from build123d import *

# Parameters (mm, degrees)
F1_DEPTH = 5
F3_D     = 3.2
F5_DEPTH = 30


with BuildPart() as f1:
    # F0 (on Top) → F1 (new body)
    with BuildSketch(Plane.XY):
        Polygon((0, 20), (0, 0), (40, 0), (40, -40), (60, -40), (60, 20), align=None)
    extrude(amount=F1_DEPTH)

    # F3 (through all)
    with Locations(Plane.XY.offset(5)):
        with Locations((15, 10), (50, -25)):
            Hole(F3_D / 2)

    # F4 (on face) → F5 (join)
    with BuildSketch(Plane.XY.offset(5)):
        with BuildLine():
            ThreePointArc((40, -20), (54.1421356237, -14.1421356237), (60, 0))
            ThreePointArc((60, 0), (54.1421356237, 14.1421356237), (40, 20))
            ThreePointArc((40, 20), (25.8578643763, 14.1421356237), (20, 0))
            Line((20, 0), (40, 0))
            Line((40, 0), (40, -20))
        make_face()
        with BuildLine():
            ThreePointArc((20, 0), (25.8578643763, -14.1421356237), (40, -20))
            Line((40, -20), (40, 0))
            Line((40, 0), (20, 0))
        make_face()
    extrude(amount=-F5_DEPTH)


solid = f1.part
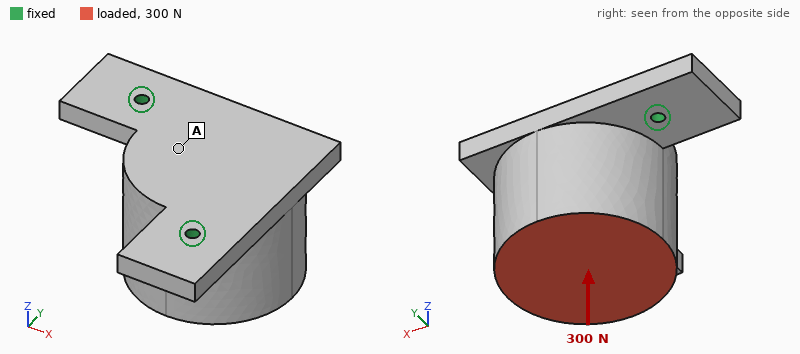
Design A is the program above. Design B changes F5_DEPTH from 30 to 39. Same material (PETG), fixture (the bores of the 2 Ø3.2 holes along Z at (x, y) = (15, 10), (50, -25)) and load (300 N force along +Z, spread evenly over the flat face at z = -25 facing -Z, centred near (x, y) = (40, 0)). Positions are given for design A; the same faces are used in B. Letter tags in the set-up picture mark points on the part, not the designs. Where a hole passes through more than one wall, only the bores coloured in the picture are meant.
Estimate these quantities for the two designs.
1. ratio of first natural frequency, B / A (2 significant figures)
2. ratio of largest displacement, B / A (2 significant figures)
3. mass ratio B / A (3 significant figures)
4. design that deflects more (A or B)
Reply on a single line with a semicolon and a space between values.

0.74; 1.1; 1.26; B
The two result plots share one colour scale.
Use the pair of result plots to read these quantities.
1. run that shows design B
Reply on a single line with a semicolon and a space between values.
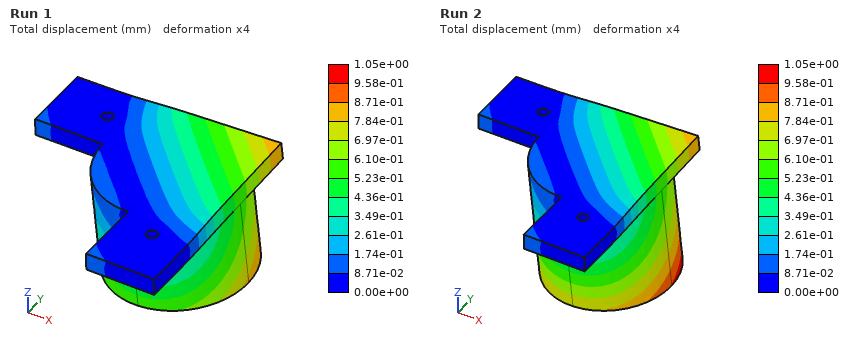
Run 2
